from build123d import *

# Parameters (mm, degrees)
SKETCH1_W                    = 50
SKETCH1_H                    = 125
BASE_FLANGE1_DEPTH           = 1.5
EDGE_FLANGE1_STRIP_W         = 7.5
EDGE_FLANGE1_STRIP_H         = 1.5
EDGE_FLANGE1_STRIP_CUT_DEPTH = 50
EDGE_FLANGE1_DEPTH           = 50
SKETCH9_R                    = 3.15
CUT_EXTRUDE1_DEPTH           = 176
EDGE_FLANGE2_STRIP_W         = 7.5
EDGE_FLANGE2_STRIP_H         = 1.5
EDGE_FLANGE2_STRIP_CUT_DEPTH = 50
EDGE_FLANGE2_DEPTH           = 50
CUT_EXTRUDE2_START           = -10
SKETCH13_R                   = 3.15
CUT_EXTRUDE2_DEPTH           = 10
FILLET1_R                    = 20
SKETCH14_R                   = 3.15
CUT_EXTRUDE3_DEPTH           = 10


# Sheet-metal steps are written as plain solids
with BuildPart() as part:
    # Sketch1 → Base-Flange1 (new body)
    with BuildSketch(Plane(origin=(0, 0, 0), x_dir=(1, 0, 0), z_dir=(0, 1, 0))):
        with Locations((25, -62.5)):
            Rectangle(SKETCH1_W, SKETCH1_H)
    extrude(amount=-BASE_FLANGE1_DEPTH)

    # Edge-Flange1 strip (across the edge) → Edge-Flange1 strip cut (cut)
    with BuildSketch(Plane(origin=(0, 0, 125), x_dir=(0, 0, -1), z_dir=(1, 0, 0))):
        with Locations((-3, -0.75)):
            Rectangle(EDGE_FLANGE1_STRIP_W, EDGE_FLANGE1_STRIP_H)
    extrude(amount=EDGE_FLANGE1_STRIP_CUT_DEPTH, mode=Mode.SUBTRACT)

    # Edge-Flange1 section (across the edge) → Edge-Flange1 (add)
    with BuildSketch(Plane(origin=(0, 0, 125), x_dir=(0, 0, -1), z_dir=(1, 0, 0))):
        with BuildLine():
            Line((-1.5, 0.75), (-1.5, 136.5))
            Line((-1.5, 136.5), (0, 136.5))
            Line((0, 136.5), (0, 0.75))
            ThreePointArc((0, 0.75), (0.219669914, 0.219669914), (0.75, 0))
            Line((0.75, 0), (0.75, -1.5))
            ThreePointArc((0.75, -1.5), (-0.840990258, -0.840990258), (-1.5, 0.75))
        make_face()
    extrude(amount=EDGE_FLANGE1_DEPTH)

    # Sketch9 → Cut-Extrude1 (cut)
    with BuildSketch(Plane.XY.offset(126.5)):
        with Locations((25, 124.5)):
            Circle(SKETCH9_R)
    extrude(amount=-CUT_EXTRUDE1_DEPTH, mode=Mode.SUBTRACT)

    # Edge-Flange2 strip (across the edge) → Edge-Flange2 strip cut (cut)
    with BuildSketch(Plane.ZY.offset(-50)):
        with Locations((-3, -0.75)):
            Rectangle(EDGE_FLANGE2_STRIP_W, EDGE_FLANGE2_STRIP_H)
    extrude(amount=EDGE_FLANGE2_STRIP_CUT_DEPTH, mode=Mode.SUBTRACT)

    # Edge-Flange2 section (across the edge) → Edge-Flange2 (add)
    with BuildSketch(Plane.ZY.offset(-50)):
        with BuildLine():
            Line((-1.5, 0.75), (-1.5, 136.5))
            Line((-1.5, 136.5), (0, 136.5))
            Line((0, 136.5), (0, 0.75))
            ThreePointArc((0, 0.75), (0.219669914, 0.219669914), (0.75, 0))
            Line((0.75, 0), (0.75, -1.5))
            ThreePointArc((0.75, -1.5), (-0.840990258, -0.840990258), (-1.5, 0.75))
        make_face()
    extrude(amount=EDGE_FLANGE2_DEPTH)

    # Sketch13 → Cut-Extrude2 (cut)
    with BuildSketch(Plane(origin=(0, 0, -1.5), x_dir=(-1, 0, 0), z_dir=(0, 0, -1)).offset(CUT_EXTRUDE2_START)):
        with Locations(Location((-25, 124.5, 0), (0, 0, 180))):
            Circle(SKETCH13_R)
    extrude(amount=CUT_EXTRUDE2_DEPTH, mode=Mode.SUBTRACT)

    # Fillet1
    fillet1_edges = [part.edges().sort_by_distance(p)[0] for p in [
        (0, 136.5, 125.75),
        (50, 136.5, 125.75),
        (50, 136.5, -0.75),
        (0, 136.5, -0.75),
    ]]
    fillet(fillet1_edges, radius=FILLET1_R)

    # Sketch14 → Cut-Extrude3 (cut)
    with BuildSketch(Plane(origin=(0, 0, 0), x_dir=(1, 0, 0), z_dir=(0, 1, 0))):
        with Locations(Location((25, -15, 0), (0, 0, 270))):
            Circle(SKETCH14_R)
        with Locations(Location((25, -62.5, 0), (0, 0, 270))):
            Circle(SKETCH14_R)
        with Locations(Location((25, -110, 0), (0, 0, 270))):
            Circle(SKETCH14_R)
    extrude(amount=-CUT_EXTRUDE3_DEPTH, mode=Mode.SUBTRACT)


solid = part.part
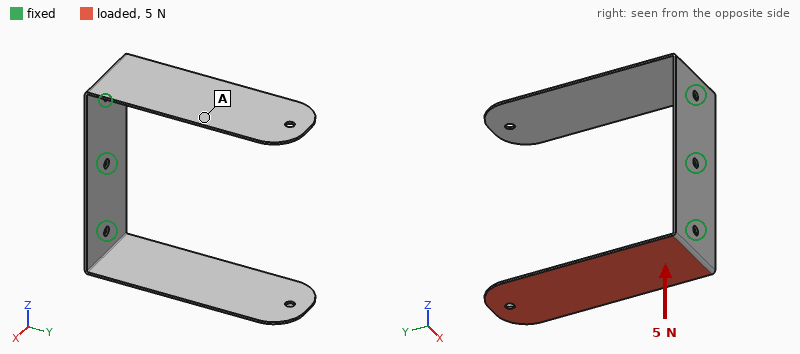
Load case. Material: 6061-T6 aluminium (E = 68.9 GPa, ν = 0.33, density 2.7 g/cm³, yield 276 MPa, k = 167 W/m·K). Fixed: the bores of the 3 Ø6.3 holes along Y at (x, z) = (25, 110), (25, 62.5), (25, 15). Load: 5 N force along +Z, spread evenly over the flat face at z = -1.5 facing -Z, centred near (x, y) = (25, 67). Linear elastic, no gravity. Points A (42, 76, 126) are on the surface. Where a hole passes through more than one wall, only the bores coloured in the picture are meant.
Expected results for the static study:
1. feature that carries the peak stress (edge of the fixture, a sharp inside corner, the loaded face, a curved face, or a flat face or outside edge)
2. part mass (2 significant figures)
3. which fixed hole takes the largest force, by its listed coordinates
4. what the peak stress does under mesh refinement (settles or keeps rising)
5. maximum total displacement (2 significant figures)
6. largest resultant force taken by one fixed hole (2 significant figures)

edge of the fixture
79 g
(25, 15)
keeps rising
2.2 mm
4.7 N
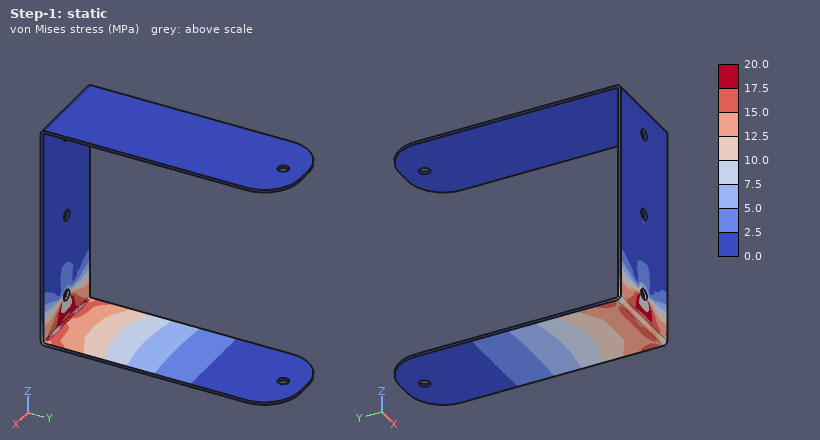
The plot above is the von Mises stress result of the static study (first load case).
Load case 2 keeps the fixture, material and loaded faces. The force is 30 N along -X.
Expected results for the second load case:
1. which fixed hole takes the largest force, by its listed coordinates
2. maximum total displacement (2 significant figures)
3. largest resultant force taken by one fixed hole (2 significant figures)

(25, 15)
2.2 mm
37 N
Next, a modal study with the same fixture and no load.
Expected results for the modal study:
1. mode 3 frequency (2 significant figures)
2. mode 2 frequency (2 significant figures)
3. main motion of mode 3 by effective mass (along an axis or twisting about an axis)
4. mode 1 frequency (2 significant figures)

140 Hz
58 Hz
along X
58 Hz
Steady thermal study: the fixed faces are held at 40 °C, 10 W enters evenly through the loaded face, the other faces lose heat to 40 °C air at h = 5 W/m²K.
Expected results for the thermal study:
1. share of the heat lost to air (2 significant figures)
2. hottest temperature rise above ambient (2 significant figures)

17 %
58 K
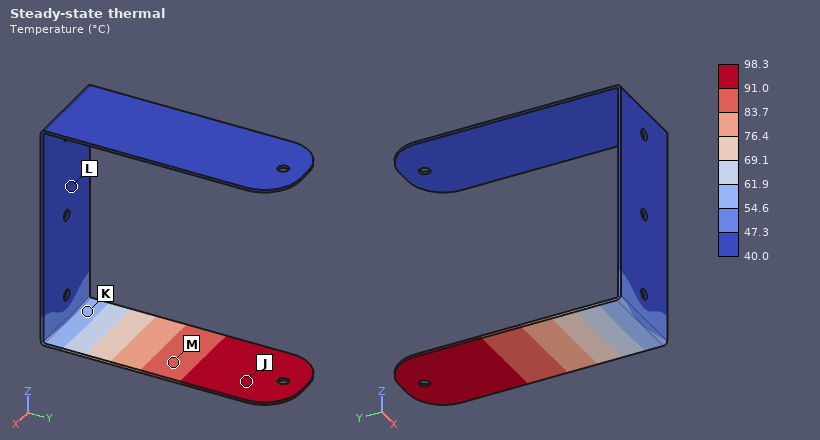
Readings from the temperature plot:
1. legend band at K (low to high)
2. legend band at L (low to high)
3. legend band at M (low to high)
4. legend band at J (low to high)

54.6 to 61.9 °C
40.0 to 47.3 °C
83.7 to 91.0 °C
91.0 to 98.3 °C
